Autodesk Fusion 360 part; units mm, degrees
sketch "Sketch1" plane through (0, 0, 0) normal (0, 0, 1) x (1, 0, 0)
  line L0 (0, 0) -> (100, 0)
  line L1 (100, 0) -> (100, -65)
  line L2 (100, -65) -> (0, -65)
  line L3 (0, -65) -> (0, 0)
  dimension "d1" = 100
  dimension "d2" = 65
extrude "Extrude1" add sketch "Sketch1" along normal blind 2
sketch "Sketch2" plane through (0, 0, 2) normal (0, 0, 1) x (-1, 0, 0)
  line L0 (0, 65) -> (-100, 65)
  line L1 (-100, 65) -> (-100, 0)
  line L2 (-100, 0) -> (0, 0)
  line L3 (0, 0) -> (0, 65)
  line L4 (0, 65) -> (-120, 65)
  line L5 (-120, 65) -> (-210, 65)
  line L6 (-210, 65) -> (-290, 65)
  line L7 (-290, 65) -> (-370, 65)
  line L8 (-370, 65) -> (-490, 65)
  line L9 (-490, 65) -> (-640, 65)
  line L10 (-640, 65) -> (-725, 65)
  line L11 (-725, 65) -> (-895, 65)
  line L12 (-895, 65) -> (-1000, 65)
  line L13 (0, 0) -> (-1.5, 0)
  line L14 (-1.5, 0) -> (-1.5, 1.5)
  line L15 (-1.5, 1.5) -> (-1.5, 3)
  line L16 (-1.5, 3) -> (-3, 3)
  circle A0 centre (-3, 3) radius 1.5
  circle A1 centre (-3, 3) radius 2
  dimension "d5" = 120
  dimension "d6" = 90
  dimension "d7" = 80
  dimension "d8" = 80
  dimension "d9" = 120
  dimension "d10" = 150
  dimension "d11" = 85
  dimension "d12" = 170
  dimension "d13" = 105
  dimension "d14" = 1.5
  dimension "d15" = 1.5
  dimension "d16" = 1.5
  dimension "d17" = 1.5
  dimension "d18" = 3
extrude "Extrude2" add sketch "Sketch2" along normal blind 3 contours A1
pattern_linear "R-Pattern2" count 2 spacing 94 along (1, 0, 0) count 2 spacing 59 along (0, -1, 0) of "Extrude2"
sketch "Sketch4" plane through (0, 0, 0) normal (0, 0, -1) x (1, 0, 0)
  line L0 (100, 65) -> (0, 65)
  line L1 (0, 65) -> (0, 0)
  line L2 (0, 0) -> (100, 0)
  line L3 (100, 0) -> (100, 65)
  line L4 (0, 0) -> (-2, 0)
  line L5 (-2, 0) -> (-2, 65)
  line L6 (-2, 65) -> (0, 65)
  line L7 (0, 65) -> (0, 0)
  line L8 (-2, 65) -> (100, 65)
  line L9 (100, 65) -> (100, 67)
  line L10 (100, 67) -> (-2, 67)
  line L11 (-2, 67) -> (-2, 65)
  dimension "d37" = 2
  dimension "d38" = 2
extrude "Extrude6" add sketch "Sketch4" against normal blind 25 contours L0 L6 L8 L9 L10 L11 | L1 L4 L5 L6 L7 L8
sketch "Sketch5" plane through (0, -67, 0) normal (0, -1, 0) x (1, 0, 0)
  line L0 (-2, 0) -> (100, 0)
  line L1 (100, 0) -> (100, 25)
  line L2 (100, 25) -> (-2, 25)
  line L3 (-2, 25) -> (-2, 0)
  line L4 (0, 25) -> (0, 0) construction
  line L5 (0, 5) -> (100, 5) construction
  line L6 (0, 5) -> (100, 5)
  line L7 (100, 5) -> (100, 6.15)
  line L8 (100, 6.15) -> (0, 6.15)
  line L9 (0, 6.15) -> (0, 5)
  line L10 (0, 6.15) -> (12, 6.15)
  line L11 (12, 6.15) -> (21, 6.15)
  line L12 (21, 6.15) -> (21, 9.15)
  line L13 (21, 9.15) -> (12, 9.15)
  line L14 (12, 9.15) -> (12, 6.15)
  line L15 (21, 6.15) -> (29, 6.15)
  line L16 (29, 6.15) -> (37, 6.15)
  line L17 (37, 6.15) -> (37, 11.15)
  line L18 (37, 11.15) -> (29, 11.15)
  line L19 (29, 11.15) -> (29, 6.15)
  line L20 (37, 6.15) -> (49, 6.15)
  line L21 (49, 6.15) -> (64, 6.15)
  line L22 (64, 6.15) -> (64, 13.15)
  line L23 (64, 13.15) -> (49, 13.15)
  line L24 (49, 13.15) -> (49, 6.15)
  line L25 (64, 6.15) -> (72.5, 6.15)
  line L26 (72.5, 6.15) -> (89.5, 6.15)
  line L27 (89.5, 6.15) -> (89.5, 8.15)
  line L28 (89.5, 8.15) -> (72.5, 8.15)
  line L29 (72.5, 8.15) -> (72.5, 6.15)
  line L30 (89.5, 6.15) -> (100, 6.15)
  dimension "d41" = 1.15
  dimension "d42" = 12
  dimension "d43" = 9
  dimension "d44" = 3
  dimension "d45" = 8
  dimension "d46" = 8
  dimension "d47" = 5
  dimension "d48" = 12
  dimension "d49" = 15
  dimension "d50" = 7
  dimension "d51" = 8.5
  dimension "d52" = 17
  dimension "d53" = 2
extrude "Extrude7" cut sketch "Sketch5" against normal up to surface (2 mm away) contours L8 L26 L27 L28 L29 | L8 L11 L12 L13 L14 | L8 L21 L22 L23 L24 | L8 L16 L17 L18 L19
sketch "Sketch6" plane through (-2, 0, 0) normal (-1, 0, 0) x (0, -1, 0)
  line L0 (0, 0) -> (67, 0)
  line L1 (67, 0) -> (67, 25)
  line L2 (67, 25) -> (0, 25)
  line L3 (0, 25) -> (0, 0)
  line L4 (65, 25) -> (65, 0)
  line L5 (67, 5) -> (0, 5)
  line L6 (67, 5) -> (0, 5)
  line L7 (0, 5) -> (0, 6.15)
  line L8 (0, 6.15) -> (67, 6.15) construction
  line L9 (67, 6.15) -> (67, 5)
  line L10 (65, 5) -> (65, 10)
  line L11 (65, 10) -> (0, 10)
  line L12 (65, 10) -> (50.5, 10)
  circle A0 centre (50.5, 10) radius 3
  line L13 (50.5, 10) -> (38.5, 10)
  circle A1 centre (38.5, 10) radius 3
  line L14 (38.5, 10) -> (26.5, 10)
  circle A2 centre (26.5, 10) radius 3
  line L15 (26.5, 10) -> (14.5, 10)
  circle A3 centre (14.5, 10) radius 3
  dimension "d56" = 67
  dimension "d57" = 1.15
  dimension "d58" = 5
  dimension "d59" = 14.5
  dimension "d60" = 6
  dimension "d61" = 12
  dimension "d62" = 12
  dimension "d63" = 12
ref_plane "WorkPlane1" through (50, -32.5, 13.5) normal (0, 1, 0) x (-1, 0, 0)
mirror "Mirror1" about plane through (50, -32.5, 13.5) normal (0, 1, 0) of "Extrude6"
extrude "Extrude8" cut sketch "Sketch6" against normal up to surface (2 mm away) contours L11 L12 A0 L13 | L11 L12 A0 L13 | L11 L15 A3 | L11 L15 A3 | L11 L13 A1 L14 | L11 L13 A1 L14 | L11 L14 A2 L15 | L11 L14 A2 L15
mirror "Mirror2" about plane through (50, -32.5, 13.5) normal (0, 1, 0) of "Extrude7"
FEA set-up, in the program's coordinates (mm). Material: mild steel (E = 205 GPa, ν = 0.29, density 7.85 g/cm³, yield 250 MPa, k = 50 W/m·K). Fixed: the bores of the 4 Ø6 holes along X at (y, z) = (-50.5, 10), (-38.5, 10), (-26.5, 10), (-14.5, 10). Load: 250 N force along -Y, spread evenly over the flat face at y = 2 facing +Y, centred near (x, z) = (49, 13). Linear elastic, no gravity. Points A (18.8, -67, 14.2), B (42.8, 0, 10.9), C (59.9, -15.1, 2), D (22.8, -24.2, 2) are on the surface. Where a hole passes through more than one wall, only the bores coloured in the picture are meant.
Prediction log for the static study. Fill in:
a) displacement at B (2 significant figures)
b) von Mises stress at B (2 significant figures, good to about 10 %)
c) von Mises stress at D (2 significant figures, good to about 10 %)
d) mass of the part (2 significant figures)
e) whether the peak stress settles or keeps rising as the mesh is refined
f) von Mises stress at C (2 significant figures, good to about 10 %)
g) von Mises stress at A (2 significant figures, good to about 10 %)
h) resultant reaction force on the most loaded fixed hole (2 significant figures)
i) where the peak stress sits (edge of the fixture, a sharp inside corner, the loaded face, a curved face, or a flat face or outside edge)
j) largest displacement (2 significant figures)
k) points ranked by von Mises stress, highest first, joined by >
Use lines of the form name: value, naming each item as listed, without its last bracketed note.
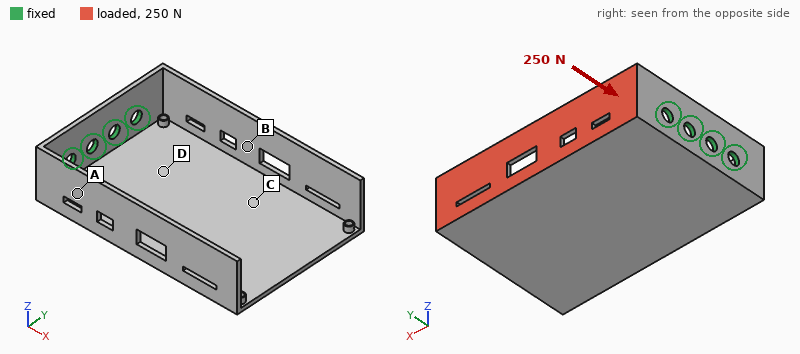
displacement at B: 0.093 mm
von Mises stress at B: 32 MPa
von Mises stress at D: 16 MPa
mass of the part: 200 g
whether the peak stress settles or keeps rising as the mesh is refined: keeps rising
von Mises stress at C: 25 MPa
von Mises stress at A: 7.0 MPa
resultant reaction force on the most loaded fixed hole: 300 N
where the peak stress sits: edge of the fixture
largest displacement: 0.31 mm
points ranked by von Mises stress, highest first, joined by >: B > C > D > A
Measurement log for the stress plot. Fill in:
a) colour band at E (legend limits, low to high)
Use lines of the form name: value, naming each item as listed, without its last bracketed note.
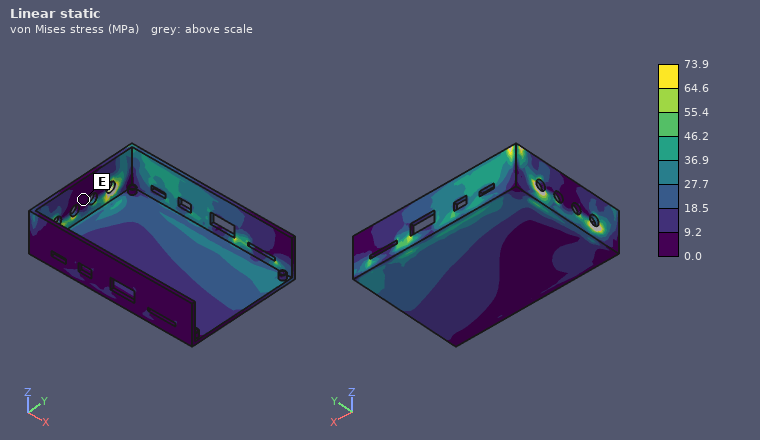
colour band at E: 0.0 to 9.2 MPa
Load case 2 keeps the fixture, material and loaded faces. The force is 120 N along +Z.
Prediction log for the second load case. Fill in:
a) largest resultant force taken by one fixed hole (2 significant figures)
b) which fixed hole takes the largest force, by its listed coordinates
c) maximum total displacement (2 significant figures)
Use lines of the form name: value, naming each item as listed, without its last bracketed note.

largest resultant force taken by one fixed hole: 200 N
which fixed hole takes the largest force, by its listed coordinates: (-14.5, 10)
maximum total displacement: 0.46 mm
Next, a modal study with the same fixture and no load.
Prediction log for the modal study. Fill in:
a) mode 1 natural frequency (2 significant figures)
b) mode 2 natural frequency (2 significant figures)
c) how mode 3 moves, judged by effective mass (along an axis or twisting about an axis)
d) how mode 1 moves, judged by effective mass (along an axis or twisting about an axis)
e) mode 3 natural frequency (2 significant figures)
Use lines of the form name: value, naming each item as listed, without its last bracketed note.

mode 1 natural frequency: 300 Hz
mode 2 natural frequency: 460 Hz
how mode 3 moves, judged by effective mass: along Y
how mode 1 moves, judged by effective mass: along Z
mode 3 natural frequency: 1100 Hz
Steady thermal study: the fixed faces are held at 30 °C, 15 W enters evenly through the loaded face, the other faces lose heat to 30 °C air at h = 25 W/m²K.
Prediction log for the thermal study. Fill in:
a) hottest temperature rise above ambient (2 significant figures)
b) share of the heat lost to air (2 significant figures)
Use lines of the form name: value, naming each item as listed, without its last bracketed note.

hottest temperature rise above ambient: 60 K
share of the heat lost to air: 64 %
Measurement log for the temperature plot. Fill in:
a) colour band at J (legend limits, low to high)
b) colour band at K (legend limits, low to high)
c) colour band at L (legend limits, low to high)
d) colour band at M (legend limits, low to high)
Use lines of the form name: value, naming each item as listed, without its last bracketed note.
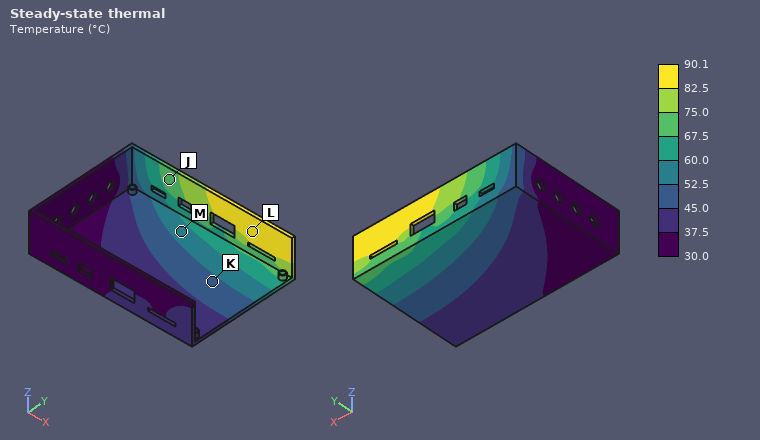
colour band at J: 67.5 to 75.0 °C
colour band at K: 45.0 to 52.5 °C
colour band at L: 82.5 to 90.1 °C
colour band at M: 52.5 to 60.0 °C
